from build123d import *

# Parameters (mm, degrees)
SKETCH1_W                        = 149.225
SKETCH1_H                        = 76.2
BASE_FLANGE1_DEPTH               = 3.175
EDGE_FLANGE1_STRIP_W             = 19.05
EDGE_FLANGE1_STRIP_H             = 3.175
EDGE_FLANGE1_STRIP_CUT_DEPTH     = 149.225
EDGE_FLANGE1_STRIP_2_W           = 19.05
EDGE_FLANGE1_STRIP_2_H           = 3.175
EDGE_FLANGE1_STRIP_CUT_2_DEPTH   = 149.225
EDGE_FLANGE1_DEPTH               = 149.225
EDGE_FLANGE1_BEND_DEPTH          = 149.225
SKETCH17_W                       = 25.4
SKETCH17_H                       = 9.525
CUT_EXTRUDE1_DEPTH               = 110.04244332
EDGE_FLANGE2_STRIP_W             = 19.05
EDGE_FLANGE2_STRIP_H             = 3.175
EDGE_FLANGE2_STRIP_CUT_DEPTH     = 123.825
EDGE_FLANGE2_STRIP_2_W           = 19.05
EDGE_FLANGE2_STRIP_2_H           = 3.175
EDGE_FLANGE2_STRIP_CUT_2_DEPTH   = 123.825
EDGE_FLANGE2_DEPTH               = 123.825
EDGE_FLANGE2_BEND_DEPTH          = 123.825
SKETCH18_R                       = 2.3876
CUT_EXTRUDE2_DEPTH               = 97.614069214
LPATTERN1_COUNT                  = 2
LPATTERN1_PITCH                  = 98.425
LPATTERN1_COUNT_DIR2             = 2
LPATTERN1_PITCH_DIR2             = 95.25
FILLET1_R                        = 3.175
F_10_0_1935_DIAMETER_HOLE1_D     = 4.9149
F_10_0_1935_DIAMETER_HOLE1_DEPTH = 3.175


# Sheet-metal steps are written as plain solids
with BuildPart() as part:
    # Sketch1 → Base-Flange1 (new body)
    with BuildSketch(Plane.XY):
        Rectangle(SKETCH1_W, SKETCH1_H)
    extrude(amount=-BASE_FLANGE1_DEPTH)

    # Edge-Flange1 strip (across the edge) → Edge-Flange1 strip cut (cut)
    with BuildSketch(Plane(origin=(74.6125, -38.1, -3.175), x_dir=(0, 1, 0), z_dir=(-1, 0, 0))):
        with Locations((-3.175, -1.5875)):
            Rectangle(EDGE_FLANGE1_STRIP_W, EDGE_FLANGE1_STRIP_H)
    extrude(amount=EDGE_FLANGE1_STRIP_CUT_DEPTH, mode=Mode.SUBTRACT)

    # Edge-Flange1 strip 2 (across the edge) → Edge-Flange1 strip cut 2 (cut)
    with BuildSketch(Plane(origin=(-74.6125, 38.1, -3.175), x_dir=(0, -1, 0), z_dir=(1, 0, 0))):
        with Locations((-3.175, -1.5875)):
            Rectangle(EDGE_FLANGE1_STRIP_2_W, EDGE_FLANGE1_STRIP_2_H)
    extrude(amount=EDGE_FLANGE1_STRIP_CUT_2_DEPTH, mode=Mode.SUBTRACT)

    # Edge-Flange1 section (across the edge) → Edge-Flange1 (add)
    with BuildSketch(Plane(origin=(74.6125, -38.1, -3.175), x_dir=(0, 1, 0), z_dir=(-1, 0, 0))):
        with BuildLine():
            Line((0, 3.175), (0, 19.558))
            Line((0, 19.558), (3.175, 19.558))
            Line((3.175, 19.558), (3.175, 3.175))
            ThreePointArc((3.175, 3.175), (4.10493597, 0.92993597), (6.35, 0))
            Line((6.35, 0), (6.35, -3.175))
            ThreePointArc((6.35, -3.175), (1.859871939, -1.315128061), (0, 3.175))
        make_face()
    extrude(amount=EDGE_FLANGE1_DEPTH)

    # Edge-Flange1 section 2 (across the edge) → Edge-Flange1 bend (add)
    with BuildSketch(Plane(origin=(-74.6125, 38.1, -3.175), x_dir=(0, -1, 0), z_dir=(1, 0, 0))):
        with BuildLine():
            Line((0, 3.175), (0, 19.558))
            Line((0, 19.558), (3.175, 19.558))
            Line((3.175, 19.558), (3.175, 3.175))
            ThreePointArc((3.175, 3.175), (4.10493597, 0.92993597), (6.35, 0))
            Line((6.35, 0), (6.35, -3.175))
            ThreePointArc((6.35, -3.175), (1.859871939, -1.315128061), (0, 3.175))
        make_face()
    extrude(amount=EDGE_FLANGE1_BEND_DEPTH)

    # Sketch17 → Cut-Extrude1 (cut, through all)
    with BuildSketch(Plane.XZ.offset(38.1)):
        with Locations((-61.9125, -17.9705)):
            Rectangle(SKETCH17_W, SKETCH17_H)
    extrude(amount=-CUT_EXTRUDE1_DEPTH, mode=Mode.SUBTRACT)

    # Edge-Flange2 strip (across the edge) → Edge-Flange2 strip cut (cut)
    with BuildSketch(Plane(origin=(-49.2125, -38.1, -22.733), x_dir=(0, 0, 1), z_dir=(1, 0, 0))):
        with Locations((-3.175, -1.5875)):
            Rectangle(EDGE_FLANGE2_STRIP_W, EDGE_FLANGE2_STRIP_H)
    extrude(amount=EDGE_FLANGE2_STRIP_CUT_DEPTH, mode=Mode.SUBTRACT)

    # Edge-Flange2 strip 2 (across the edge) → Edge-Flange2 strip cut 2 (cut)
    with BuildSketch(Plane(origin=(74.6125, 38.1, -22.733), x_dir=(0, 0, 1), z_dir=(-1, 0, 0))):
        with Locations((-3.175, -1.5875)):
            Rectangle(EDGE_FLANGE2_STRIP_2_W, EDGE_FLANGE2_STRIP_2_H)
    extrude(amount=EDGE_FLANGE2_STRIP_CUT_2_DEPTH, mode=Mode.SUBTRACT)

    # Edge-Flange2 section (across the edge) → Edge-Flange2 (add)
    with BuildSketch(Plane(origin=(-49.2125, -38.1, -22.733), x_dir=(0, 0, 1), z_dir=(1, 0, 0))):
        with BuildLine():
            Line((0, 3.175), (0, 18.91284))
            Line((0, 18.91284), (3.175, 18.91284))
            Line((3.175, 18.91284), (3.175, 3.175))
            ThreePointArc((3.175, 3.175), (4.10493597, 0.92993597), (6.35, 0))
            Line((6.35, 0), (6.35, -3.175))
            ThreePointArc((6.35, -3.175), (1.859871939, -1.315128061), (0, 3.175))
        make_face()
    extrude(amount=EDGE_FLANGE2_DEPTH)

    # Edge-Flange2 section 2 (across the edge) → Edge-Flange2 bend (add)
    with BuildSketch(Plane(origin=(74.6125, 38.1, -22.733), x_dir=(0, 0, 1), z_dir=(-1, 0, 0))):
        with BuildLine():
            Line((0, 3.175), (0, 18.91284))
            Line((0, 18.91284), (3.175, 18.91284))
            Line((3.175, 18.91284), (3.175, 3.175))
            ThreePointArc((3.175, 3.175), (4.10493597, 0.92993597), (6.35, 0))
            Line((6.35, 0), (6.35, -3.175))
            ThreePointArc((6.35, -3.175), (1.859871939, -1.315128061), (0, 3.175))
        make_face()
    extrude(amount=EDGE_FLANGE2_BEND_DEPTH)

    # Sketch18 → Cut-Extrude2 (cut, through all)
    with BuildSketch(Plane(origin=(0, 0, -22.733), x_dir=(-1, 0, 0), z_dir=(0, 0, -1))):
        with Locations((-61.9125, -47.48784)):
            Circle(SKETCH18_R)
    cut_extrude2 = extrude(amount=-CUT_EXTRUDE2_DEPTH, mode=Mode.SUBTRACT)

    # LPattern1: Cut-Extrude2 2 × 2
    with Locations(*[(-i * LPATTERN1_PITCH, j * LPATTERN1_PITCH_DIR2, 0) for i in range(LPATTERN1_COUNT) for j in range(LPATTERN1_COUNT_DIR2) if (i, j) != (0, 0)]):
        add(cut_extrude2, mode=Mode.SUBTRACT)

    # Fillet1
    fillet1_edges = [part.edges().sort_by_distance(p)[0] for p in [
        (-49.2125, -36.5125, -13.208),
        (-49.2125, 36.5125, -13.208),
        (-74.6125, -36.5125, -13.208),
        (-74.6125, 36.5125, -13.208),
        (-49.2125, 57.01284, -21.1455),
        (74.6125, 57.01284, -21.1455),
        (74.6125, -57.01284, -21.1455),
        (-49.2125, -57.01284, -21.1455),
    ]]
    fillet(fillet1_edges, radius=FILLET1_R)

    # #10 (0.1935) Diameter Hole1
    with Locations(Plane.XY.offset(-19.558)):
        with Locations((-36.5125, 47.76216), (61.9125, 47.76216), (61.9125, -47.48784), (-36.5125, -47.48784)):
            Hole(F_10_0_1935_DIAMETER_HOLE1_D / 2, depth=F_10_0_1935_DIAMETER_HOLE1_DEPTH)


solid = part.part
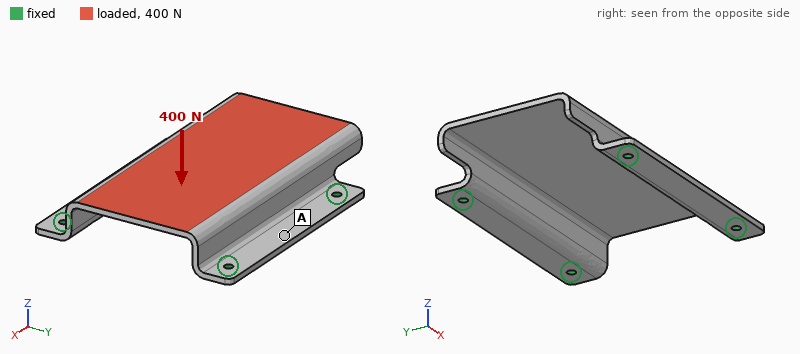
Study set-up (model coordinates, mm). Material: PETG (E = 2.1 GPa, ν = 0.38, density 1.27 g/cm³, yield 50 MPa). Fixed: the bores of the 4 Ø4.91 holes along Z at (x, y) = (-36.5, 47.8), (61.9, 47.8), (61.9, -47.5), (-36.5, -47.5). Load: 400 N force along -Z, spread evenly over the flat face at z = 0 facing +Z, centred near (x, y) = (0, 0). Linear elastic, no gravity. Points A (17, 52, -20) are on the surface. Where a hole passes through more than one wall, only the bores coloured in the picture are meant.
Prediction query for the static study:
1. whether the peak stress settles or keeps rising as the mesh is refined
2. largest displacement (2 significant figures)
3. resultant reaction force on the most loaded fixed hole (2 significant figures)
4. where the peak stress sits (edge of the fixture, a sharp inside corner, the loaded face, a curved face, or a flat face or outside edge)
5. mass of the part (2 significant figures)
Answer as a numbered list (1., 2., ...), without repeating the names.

1. keeps rising
2. 1.3 mm
3. 170 N
4. edge of the fixture
5. 81 g
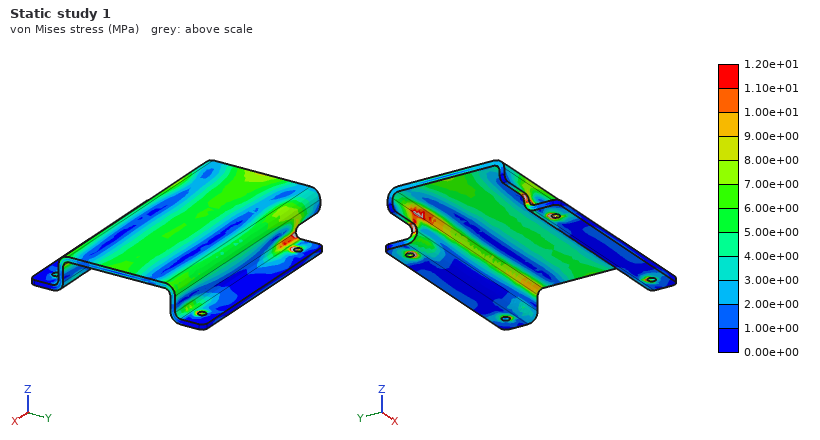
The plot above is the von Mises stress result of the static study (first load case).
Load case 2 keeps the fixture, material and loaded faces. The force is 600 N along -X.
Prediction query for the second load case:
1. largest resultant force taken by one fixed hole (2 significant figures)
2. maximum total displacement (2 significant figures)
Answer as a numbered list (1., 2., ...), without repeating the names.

1. 170 N
2. 0.36 mm
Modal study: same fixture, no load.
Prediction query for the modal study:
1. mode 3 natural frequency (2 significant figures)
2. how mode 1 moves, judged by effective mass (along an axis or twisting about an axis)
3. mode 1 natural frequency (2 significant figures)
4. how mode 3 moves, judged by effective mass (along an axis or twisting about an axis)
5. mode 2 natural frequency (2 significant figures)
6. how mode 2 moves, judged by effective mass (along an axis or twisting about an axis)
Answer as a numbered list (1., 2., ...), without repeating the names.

1. 680 Hz
2. along Y
3. 500 Hz
4. along Z
5. 580 Hz
6. along Z
